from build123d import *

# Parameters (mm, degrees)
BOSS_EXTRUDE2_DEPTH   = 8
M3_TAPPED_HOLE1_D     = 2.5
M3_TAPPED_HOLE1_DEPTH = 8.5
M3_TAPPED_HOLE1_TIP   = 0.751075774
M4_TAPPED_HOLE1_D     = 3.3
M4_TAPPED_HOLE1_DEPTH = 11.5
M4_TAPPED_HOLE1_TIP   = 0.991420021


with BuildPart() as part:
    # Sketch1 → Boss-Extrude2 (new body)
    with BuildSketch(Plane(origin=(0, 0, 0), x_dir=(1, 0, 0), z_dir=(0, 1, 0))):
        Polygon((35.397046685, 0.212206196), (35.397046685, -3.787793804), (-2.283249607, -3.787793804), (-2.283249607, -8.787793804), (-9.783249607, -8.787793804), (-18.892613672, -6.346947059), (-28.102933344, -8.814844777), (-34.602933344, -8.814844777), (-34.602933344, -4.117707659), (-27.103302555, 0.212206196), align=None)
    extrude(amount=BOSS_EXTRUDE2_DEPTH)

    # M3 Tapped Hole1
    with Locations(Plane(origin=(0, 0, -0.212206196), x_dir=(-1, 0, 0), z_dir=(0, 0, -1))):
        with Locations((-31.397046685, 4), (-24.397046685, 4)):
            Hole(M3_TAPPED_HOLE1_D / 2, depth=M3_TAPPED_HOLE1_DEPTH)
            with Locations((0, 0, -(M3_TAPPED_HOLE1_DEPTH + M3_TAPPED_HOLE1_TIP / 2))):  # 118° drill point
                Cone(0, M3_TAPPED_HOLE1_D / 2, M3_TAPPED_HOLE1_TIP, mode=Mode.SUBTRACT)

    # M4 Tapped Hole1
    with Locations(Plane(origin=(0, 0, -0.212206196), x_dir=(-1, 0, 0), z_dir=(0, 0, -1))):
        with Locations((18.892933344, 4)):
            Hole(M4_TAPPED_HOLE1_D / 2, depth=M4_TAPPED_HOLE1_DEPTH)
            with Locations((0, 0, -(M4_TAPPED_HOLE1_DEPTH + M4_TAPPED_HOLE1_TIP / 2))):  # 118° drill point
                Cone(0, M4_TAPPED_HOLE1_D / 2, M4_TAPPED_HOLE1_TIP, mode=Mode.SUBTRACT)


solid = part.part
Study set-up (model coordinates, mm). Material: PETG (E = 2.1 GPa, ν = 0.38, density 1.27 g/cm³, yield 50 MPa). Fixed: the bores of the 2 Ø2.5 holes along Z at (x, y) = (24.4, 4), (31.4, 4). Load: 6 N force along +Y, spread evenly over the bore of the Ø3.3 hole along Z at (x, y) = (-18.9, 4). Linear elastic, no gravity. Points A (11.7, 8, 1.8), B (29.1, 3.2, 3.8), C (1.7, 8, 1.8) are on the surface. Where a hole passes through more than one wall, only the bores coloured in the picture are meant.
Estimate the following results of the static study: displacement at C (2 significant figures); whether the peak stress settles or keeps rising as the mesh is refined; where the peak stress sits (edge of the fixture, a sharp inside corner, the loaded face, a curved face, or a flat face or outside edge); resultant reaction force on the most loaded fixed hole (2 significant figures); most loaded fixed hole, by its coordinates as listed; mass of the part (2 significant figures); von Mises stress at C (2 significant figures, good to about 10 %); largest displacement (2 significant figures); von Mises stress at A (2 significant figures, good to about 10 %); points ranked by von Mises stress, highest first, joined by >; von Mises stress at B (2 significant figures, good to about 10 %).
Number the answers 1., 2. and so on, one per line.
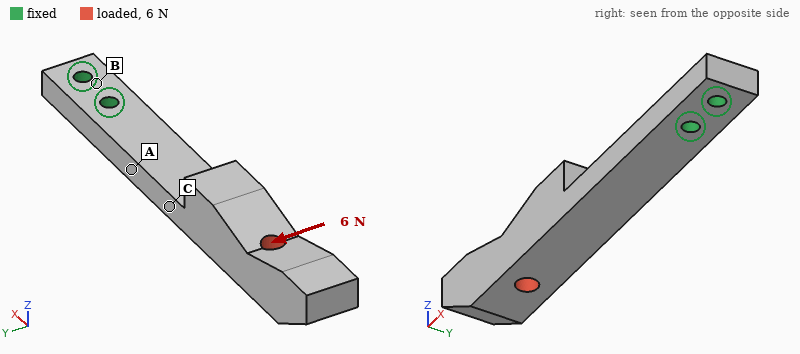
1. 0.21 mm
2. keeps rising
3. edge of the fixture
4. 24 N
5. (24.4, 4)
6. 4.0 g
7. 3.0 MPa
8. 0.81 mm
9. 4.3 MPa
10. A > C > B
11. 1.3 MPa
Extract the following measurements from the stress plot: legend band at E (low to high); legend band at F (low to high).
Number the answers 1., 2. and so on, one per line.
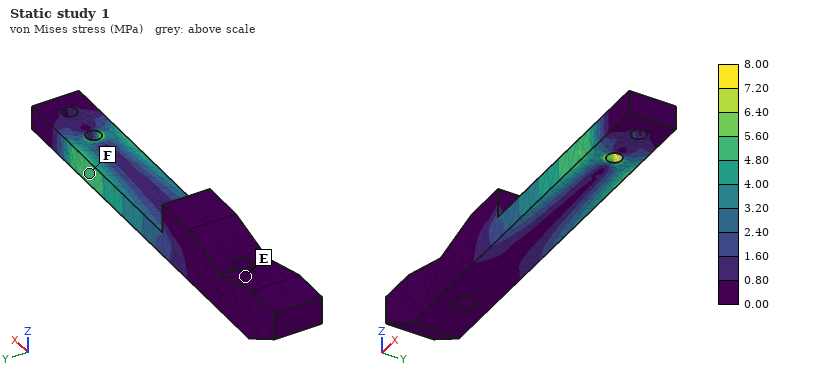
1. 0.00 to 0.80 MPa
2. 4.80 to 5.60 MPa
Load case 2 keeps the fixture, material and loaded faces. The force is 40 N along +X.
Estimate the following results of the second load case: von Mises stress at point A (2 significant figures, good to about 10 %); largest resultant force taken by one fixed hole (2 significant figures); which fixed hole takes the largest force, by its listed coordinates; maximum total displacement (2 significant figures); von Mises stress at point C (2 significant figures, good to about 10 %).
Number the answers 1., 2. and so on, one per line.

1. 1.3 MPa
2. 35 N
3. (24.4, 4)
4. 0.79 mm
5. 1.2 MPa
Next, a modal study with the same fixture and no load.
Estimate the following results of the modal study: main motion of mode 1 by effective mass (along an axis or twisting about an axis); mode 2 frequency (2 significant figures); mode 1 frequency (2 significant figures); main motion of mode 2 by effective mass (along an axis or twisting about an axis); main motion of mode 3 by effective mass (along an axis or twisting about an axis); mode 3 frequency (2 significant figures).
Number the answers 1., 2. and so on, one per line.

1. along Z
2. 330 Hz
3. 190 Hz
4. along Y
5. along Z
6. 1500 Hz
